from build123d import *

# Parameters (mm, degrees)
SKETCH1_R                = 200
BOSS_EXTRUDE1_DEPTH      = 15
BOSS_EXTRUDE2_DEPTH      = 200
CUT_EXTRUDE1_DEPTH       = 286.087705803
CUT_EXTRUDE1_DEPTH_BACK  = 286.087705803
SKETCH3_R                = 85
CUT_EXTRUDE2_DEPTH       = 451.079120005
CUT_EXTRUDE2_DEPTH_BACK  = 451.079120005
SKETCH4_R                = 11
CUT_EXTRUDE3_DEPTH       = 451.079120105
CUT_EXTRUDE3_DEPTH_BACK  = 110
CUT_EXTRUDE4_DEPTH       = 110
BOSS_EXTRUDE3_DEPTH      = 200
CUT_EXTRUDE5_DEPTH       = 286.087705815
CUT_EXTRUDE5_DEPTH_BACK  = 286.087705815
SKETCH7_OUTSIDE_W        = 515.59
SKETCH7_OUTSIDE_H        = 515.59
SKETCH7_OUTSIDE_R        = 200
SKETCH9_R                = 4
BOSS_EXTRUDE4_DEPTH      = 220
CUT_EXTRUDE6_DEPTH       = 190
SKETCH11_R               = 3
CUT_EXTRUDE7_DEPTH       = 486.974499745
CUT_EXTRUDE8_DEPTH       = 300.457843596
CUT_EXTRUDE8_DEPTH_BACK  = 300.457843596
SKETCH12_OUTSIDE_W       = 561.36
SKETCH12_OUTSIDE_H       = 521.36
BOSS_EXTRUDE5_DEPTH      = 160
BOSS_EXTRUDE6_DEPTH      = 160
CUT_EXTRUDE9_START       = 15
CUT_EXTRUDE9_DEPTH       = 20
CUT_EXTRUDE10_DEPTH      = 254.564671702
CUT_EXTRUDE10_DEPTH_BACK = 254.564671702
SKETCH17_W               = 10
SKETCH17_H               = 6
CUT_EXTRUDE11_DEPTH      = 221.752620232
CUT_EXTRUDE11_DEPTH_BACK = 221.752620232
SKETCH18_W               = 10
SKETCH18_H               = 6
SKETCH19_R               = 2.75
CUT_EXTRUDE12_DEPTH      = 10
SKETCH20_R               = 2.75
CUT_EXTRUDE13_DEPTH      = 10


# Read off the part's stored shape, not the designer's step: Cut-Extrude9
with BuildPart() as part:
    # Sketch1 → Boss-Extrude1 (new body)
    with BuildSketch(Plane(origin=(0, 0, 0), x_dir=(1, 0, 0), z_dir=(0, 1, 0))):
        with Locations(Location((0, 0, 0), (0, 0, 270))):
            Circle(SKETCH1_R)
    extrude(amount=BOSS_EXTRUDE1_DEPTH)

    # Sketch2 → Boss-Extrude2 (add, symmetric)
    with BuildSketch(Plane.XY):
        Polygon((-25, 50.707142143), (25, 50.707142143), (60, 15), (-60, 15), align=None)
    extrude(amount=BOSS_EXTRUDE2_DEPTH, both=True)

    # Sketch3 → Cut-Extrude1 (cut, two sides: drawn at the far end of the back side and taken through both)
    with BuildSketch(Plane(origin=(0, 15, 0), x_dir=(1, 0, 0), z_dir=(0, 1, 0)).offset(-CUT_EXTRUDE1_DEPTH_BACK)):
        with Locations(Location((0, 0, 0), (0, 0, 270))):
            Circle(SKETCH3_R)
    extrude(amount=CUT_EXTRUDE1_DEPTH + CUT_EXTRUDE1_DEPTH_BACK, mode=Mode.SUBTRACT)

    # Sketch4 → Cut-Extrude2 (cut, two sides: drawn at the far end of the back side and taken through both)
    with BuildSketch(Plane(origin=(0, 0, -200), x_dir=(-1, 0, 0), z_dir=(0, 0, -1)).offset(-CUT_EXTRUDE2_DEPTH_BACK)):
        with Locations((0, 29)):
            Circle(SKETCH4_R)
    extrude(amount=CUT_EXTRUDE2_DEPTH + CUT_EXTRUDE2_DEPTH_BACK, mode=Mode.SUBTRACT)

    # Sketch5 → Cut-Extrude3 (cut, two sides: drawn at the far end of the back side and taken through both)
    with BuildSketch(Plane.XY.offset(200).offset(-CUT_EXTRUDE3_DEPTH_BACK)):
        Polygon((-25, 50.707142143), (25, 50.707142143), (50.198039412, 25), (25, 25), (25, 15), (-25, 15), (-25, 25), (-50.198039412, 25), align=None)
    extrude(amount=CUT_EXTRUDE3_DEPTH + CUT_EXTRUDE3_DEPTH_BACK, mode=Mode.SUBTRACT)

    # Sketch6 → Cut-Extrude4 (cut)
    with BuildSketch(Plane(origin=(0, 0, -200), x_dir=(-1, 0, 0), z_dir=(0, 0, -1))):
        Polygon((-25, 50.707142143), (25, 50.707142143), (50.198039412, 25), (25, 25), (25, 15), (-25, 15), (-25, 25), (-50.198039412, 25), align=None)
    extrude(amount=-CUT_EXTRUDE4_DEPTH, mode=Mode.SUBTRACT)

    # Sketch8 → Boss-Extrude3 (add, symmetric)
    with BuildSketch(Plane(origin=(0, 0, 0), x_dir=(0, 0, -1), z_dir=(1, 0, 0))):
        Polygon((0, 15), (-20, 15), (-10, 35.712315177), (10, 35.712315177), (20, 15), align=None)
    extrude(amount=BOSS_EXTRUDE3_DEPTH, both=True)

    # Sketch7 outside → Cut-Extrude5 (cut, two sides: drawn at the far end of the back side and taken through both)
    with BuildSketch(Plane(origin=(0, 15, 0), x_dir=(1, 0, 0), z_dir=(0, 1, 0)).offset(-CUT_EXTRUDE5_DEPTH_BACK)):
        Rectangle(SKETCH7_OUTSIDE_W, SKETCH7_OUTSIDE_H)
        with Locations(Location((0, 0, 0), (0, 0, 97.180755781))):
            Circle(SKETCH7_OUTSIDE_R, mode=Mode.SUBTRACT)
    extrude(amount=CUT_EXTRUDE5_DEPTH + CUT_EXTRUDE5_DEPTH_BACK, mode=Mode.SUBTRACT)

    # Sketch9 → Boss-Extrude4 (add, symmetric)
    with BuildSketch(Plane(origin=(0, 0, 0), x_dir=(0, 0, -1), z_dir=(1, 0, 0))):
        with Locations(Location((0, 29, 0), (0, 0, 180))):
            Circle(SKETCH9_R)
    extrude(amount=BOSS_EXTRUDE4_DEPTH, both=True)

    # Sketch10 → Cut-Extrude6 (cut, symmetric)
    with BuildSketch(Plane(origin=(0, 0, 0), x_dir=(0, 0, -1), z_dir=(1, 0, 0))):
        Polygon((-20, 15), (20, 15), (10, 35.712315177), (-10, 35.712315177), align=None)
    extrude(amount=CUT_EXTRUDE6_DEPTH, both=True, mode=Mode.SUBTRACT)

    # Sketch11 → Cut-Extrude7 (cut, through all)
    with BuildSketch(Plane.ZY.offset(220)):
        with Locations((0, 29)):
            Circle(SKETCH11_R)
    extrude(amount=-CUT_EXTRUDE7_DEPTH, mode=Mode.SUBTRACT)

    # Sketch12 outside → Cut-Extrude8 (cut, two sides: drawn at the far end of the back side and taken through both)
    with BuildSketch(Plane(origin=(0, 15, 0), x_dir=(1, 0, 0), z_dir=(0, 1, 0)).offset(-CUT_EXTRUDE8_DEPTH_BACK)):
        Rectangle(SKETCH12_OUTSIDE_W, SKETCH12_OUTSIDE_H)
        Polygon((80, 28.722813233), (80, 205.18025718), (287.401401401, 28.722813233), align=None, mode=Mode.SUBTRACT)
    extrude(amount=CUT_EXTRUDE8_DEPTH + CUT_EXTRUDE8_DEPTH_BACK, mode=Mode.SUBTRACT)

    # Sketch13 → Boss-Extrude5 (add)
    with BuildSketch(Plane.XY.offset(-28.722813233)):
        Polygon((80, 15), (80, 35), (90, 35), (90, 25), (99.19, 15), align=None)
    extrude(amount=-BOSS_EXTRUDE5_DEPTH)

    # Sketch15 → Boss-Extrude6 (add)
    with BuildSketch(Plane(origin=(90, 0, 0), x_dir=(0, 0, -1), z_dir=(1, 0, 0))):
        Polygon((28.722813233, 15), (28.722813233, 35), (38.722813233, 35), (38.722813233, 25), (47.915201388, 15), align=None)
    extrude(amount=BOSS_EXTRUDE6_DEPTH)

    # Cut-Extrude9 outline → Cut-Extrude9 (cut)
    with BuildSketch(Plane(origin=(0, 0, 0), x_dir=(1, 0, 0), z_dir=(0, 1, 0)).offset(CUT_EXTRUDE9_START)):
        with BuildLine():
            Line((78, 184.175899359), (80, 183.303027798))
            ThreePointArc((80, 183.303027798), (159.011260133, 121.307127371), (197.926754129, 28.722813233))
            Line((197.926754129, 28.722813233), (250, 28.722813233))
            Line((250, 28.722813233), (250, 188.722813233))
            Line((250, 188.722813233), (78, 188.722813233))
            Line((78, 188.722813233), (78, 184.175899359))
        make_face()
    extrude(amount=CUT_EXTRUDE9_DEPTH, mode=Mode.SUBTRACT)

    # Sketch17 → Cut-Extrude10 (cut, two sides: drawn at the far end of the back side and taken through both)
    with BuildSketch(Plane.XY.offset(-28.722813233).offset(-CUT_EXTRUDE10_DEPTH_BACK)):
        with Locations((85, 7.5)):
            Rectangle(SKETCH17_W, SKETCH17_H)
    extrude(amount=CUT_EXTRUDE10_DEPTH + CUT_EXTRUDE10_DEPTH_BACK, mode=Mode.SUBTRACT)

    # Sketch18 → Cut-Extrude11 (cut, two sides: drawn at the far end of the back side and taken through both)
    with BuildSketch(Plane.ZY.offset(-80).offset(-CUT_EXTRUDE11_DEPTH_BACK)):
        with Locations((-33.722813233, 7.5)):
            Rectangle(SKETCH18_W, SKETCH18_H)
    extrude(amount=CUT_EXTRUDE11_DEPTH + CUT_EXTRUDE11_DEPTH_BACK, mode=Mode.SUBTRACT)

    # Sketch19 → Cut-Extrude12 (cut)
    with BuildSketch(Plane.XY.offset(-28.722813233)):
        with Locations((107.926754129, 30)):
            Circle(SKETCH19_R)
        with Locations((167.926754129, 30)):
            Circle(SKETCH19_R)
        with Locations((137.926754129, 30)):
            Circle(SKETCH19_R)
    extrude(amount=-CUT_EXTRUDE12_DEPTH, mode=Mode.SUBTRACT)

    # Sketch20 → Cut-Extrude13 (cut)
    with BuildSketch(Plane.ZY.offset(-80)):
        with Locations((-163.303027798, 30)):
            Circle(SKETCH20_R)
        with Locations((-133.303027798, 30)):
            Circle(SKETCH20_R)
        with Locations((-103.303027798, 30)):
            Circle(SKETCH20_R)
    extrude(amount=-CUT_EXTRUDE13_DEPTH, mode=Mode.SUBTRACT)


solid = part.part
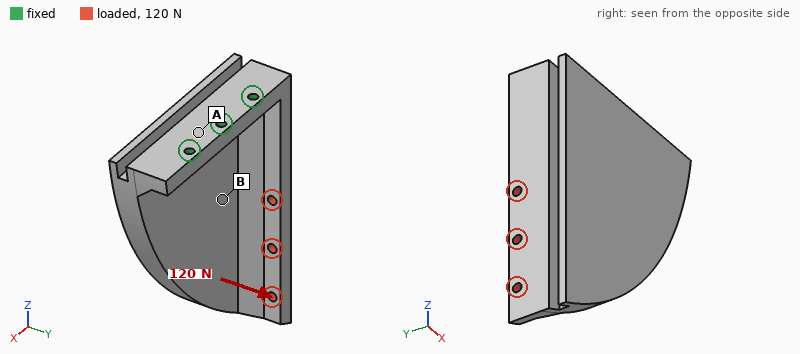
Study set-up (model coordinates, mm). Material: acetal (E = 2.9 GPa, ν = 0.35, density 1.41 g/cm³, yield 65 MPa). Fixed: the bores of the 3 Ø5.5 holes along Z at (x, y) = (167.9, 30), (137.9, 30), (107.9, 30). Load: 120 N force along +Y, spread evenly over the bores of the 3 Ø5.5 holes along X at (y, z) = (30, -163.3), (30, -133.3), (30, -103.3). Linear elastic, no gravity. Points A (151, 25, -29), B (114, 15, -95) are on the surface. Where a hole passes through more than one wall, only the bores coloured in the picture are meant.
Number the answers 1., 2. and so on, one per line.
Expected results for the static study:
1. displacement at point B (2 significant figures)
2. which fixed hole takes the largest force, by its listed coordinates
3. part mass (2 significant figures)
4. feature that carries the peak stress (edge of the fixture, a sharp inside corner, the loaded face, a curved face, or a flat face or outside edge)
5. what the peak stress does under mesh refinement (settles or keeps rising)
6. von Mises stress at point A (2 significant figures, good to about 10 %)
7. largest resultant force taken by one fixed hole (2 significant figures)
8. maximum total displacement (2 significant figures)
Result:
1. 0.68 mm
2. (107.9, 30)
3. 330 g
4. edge of the fixture
5. keeps rising
6. 3.1 MPa
7. 140 N
8. 2.0 mm
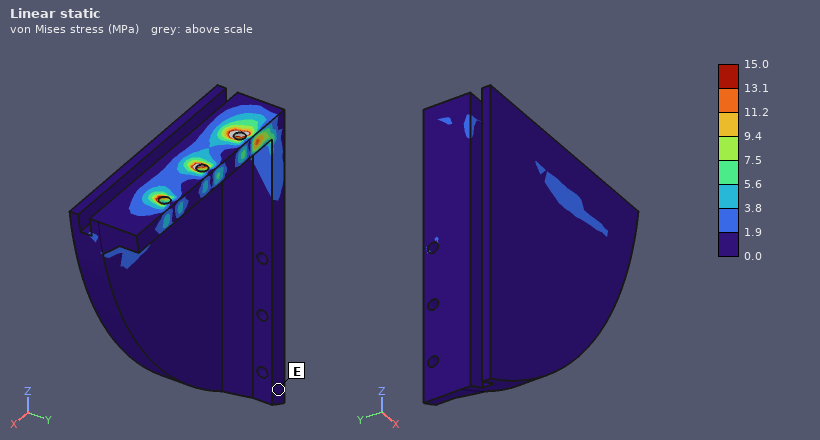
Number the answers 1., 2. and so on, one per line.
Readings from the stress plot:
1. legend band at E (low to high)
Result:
1. 0.0 to 1.9 MPa
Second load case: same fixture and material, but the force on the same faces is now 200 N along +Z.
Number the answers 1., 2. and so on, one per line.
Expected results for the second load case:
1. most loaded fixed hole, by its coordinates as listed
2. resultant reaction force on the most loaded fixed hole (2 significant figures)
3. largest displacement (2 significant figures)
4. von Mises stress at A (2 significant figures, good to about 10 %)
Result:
1. (107.9, 30)
2. 240 N
3. 0.29 mm
4. 0.62 MPa
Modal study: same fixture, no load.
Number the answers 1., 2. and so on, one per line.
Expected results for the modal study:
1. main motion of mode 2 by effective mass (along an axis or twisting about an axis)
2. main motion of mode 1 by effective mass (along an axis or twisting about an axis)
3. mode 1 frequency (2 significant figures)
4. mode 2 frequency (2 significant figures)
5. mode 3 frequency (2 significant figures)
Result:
1. along X
2. along Y
3. 130 Hz
4. 370 Hz
5. 680 Hz
